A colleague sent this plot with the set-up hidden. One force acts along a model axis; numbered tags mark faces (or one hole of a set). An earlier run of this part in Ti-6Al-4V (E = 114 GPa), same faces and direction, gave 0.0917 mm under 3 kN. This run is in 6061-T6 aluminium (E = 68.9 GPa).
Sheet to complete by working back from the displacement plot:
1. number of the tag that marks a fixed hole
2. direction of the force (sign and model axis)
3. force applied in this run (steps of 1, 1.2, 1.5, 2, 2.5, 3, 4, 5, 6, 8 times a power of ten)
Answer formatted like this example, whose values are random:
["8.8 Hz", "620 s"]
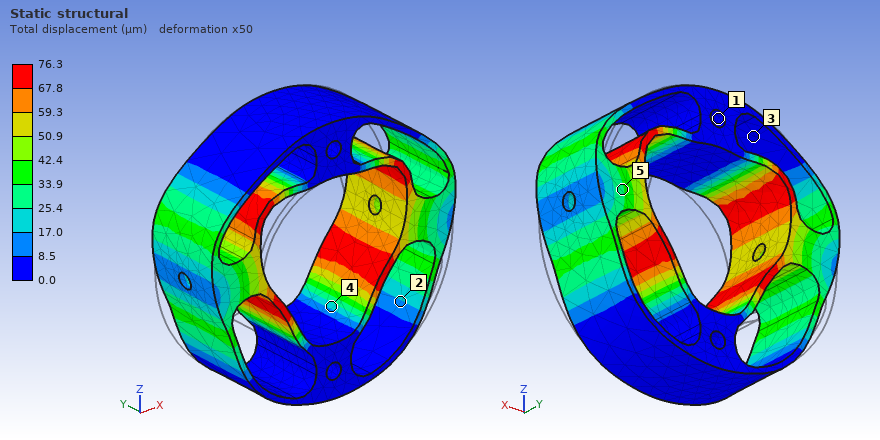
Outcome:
["1", "+Z", "1.5 kN"]
